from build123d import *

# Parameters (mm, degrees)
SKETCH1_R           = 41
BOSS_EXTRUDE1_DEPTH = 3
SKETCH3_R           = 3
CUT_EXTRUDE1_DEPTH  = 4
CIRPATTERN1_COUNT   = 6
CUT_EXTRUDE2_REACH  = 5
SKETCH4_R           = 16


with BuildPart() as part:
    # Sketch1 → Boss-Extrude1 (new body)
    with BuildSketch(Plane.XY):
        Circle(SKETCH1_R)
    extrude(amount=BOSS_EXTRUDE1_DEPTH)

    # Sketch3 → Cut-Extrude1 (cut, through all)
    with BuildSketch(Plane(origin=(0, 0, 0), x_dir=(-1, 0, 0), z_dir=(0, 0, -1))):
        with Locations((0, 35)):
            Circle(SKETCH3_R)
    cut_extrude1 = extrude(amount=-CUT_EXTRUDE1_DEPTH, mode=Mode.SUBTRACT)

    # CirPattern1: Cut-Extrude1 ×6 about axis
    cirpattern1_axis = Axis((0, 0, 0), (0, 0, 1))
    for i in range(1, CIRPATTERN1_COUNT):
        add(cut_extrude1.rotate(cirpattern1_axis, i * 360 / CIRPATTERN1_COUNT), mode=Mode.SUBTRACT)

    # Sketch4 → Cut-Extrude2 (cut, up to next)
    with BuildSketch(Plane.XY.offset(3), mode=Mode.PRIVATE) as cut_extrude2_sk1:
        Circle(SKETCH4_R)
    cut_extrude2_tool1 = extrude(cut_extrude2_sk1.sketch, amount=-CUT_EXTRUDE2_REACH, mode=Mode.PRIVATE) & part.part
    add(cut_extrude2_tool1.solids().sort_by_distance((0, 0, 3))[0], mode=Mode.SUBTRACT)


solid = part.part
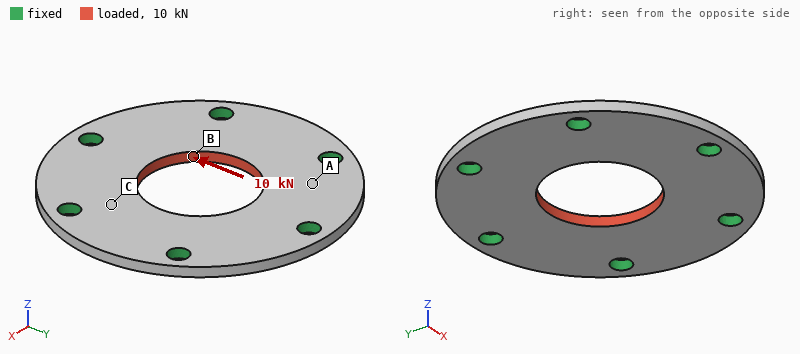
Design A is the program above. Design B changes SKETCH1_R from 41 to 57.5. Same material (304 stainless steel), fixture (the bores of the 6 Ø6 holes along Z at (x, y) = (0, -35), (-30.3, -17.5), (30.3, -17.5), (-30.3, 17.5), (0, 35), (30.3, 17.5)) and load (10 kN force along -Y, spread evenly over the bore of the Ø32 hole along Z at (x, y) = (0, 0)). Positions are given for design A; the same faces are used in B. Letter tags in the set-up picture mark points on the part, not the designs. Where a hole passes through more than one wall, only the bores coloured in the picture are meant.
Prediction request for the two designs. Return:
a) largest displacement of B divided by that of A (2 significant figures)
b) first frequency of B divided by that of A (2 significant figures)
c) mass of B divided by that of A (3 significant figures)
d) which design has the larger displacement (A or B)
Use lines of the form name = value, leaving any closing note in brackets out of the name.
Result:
largest displacement of B divided by that of A = 0.89
first frequency of B divided by that of A = 0.49
mass of B divided by that of A = 2.19
which design has the larger displacement = A
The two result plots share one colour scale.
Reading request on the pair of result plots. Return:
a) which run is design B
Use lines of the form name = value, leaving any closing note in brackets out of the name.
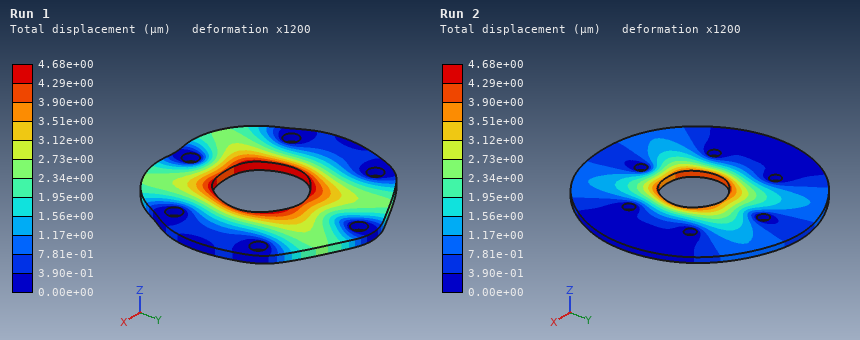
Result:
which run is design B = Run 2
